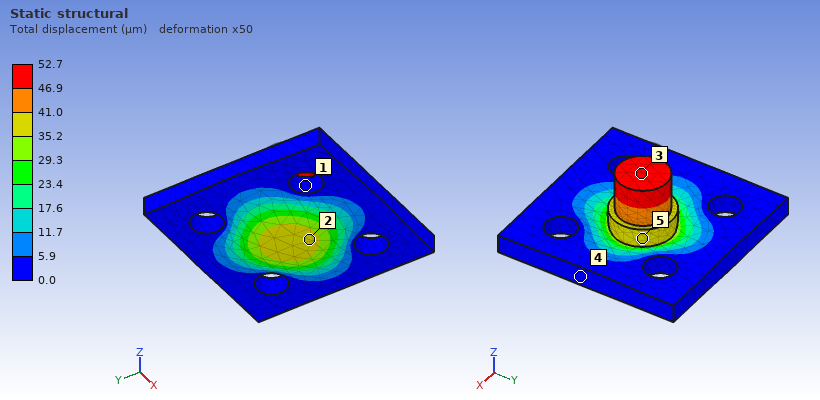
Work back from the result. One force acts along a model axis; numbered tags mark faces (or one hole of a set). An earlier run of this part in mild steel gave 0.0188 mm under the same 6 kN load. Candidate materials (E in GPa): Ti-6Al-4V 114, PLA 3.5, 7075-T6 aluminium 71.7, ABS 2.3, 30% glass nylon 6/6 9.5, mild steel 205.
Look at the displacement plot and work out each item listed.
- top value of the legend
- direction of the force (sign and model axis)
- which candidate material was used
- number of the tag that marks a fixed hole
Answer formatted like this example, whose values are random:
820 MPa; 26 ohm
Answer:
52.7 µm; -Z; 7075-T6 aluminium; 1
